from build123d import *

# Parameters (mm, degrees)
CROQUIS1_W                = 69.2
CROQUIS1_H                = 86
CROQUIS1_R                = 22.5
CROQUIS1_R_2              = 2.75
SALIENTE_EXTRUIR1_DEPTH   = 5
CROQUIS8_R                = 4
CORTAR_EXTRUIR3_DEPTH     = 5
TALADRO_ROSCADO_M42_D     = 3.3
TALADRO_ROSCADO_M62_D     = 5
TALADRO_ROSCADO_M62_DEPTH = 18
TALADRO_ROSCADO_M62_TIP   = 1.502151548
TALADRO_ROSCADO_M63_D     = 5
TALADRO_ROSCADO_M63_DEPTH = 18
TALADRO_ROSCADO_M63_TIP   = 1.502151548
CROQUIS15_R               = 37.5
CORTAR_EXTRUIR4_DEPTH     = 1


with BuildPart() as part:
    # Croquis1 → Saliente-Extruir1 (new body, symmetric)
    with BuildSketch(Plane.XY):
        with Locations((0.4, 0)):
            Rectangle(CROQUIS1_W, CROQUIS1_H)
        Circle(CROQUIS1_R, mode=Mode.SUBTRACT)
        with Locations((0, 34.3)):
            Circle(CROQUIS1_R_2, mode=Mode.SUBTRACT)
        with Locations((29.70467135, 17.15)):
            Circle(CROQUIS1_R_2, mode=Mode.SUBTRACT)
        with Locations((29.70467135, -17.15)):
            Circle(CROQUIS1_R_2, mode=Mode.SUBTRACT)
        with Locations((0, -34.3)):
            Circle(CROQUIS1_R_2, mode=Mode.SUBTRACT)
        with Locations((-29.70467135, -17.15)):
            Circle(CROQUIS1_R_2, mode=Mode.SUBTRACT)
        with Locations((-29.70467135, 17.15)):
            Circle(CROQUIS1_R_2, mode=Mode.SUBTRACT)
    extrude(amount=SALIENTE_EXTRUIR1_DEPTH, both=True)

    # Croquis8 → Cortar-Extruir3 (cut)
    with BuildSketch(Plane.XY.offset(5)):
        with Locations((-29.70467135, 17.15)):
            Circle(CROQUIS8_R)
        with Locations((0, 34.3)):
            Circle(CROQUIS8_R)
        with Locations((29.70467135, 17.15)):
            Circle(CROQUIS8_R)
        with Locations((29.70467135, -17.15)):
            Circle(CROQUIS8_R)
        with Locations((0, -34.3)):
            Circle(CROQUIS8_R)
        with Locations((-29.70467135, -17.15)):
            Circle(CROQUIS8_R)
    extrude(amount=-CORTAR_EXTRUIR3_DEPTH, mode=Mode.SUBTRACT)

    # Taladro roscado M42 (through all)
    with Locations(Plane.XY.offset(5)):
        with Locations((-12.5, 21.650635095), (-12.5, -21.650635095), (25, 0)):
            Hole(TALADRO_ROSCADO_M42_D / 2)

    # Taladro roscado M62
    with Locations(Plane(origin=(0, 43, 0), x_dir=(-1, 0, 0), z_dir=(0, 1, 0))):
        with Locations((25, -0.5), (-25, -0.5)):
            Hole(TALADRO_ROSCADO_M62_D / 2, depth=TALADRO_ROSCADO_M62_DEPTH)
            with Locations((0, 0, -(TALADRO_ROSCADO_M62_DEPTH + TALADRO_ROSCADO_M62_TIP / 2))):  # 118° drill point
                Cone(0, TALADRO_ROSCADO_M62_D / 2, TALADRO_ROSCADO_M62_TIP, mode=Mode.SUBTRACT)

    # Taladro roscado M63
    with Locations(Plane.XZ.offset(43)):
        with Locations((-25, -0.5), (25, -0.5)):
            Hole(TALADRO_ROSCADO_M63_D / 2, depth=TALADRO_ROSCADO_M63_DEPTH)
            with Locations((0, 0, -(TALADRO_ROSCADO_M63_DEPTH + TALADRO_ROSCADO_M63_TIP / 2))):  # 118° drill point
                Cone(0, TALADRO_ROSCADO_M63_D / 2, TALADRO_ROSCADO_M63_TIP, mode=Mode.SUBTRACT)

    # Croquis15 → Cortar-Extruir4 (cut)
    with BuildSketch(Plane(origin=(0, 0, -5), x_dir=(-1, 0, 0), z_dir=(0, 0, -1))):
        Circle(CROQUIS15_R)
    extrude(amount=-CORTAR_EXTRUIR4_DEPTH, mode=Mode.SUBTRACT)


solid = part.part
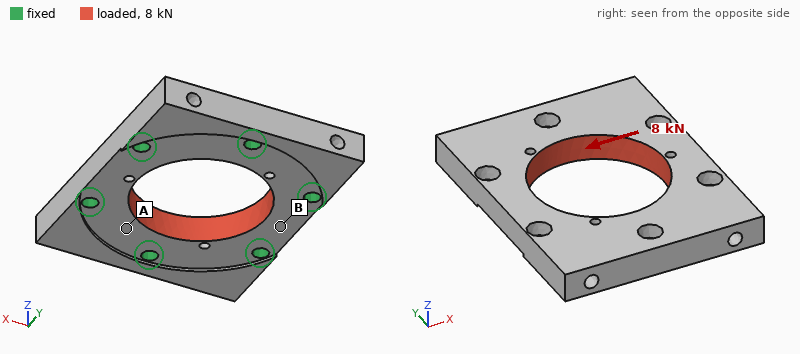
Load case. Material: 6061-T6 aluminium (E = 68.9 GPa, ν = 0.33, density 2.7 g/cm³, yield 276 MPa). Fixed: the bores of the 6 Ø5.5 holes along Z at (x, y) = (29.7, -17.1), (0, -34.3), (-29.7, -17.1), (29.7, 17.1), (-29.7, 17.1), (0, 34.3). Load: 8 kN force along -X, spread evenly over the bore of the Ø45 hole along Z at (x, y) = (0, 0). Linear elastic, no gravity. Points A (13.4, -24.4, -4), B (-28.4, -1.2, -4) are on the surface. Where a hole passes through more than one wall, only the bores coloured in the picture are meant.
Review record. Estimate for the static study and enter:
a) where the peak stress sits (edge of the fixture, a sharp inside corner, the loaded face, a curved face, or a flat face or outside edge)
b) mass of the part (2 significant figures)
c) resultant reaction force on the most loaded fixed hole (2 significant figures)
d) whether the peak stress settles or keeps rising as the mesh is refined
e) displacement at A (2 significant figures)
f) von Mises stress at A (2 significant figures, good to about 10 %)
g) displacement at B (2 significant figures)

edge of the fixture
100 g
1.4 kN
keeps rising
2.3 µm
10 MPa
4.7 µm
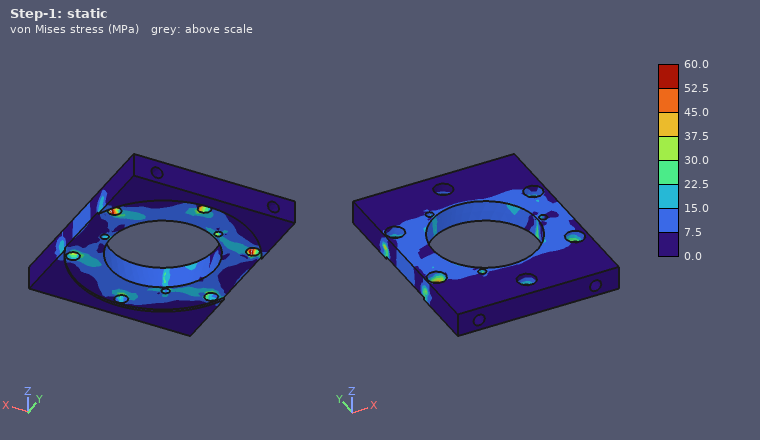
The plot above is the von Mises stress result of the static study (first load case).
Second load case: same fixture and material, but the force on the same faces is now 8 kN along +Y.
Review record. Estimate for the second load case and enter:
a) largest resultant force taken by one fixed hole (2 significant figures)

1.5 kN
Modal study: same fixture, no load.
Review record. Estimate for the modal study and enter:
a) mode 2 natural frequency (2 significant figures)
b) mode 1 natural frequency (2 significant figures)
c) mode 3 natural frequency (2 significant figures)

11 kHz
11 kHz
11 kHz
